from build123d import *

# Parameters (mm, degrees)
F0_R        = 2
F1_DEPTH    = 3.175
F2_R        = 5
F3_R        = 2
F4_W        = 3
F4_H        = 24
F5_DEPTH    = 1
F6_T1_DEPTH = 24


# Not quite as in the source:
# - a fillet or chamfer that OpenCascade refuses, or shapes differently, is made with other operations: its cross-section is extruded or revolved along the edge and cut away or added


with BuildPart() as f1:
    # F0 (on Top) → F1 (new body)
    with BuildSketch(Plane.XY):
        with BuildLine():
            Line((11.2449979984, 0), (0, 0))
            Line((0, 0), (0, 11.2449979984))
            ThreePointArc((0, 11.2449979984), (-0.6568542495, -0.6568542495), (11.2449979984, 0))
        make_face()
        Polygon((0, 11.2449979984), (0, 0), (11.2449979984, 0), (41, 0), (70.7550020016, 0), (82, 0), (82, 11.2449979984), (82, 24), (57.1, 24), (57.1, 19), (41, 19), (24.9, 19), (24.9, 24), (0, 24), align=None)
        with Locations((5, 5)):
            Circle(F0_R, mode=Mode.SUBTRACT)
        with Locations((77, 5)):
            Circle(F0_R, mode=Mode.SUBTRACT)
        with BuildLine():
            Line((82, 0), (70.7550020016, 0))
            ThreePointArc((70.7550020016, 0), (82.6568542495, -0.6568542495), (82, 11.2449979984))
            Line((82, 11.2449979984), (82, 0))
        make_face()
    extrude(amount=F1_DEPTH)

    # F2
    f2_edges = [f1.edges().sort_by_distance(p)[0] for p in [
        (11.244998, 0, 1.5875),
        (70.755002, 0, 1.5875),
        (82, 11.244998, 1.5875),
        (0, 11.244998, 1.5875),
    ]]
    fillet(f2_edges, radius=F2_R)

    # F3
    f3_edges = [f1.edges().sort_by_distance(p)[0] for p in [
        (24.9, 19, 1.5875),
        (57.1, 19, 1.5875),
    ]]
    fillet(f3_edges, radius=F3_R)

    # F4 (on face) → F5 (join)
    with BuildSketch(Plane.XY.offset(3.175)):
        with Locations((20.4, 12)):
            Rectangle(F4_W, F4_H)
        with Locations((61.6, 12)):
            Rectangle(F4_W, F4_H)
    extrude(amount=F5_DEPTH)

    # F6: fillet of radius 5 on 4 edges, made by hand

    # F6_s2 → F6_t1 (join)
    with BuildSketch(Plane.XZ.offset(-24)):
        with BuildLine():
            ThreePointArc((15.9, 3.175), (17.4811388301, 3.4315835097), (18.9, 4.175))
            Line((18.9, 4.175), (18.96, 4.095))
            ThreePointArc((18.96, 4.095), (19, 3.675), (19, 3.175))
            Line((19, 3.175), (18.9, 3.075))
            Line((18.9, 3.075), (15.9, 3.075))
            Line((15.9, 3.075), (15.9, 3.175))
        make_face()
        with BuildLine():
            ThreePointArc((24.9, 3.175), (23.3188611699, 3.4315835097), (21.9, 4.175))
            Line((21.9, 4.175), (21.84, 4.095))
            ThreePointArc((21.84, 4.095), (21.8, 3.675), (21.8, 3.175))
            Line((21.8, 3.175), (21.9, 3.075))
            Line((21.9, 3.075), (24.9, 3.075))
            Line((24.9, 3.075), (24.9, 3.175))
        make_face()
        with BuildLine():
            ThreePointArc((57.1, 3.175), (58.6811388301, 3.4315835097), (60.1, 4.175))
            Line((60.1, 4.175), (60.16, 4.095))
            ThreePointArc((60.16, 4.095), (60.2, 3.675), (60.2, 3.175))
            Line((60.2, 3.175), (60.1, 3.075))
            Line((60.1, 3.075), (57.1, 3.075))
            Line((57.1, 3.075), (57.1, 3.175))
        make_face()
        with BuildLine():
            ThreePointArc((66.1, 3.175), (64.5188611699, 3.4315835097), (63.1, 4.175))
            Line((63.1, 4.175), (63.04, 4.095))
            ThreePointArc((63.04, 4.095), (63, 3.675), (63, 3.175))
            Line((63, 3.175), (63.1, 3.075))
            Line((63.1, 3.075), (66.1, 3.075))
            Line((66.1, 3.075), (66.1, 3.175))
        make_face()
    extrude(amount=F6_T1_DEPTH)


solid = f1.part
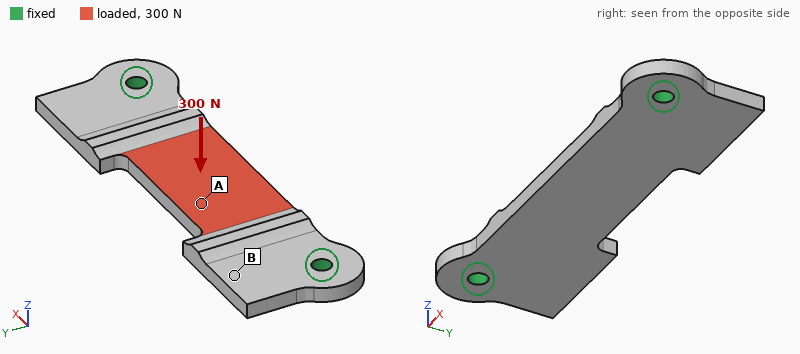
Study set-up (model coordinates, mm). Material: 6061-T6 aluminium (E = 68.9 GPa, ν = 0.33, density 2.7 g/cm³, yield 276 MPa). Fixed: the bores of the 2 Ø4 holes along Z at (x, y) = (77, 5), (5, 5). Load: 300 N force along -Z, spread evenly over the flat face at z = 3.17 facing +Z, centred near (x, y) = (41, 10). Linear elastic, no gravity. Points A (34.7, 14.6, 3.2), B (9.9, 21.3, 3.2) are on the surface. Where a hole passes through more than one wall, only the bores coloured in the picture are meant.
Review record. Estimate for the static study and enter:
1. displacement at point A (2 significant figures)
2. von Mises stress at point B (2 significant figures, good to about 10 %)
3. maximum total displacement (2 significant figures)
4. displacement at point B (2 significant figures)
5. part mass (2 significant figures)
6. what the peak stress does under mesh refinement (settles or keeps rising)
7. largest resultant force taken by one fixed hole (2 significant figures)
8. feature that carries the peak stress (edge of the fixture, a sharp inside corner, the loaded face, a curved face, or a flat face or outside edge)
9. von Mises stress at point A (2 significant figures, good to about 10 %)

0.14 mm
21 MPa
0.16 mm
0.027 mm
17 g
keeps rising
150 N
edge of the fixture
43 MPa
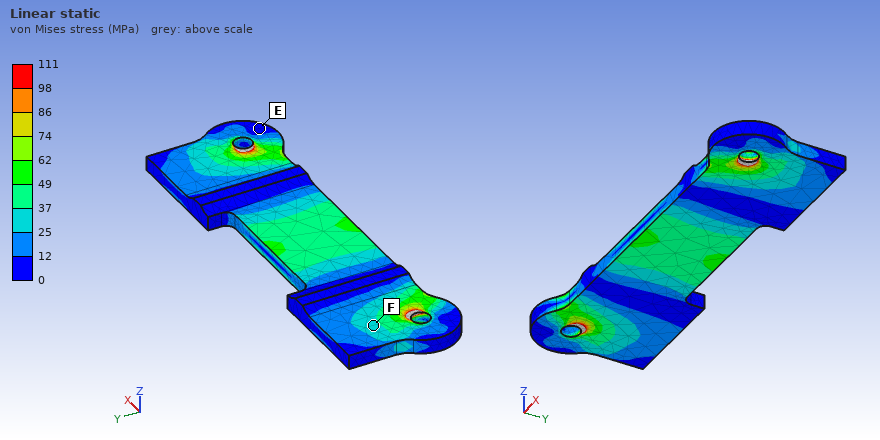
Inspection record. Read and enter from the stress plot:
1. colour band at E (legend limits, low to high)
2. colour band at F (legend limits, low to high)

0 to 12 MPa
25 to 37 MPa
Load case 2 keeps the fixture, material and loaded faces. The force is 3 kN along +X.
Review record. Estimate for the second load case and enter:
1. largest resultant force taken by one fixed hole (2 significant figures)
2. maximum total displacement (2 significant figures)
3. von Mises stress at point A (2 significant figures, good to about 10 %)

1.5 kN
26 µm
22 MPa
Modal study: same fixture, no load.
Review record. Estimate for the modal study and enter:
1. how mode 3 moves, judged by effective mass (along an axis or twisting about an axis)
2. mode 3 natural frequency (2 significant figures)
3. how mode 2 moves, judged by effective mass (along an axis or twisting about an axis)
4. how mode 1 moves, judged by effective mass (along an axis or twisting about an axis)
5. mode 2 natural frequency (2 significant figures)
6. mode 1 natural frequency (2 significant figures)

twisting about Y
6300 Hz
twisting about X
along Z
5600 Hz
2900 Hz
